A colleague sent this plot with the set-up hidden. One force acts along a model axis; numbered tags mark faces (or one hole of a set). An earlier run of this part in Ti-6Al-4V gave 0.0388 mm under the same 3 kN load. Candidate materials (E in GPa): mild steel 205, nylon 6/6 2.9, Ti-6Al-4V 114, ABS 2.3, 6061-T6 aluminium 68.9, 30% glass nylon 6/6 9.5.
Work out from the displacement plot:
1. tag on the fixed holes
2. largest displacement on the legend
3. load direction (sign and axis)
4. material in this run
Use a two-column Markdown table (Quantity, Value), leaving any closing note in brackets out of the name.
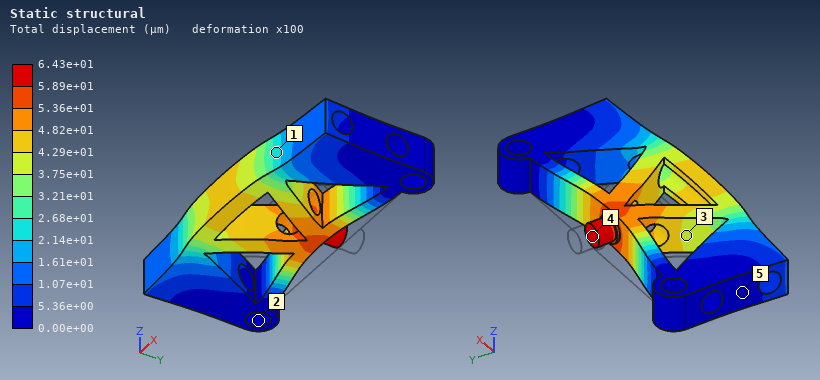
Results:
| Quantity | Value |
|---|---|
| tag on the fixed holes | 2 |
| largest displacement on the legend | 6.43e+01 µm |
| load direction | -Y |
| material in this run | 6061-T6 aluminium |
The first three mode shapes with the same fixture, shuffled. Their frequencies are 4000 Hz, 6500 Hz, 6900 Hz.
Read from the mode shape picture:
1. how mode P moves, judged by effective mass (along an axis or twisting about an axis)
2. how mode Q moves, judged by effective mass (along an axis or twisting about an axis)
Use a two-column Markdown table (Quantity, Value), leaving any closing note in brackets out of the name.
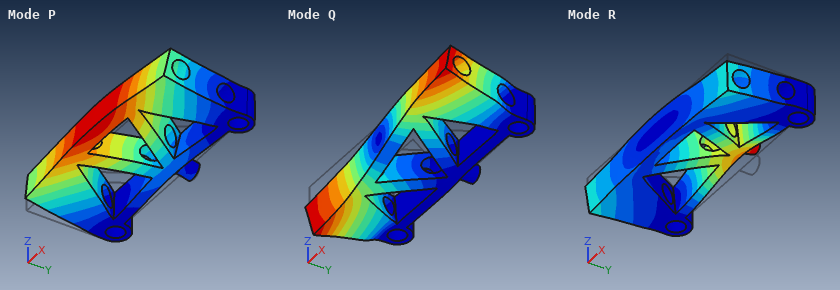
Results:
| Quantity | Value |
|---|---|
| how mode P moves, judged by effective mass | along Z |
| how mode Q moves, judged by effective mass | twisting about Y |
